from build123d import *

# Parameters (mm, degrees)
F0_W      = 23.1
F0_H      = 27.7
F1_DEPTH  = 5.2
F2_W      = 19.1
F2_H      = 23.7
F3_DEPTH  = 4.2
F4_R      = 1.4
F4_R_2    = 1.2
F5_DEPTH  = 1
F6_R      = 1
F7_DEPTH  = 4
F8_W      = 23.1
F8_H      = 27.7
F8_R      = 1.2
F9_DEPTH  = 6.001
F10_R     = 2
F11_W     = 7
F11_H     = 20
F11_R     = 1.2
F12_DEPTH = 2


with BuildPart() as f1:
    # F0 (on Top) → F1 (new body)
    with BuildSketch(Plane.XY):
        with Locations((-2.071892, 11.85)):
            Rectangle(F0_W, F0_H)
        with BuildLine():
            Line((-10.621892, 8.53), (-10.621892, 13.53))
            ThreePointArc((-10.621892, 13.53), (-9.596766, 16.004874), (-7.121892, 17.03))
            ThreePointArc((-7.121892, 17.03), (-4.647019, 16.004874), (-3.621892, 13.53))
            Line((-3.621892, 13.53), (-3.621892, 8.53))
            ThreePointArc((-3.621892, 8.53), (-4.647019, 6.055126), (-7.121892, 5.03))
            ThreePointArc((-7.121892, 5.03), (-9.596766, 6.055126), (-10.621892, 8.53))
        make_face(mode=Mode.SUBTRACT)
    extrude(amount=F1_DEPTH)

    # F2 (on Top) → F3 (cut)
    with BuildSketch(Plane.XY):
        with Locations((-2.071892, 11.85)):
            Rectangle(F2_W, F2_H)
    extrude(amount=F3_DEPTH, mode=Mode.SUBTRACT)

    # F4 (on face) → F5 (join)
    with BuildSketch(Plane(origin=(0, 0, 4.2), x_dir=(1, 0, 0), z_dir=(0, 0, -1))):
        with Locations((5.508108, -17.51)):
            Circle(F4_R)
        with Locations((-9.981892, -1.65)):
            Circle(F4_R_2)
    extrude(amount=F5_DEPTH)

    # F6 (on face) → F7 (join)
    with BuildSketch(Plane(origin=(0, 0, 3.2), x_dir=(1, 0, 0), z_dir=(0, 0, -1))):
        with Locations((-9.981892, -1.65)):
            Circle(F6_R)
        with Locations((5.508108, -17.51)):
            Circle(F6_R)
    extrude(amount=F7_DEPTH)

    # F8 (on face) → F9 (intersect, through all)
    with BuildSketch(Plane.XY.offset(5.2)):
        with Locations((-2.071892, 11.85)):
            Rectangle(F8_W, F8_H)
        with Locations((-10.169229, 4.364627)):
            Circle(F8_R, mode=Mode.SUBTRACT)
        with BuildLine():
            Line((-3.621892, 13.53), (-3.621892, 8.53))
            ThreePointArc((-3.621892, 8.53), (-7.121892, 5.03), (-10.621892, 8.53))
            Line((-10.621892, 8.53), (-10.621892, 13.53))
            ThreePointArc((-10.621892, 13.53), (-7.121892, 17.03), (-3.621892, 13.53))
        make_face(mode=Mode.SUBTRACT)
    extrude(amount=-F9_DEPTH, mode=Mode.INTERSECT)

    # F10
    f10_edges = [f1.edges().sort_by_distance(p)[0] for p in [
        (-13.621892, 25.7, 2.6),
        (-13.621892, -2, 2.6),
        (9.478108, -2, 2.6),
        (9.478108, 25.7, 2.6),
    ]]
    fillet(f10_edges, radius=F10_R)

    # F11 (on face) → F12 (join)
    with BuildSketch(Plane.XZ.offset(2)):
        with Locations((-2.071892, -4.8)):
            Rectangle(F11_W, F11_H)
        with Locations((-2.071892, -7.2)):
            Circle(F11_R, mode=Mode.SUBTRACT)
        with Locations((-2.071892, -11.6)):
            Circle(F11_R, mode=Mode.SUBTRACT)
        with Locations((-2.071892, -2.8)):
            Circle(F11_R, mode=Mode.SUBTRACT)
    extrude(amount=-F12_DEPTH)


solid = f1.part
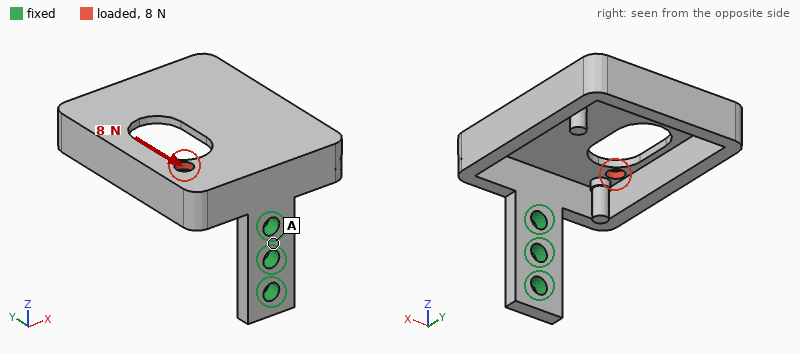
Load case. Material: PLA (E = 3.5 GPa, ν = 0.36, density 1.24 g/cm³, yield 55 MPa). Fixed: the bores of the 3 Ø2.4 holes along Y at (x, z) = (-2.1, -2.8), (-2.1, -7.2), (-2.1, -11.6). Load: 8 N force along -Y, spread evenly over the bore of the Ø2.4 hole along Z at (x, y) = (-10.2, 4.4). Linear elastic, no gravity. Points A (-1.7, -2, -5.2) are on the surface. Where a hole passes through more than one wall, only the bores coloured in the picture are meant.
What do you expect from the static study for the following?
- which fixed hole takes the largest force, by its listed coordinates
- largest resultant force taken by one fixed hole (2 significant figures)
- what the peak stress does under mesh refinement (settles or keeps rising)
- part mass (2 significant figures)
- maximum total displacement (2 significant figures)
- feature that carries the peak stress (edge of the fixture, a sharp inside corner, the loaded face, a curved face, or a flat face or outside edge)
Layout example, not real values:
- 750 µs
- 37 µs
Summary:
- (-2.1, -2.8)
- 10.0 N
- keeps rising
- 1.9 g
- 0.49 mm
- edge of the fixture
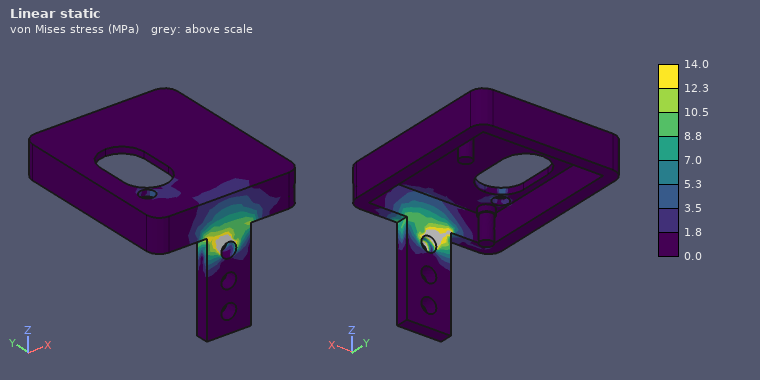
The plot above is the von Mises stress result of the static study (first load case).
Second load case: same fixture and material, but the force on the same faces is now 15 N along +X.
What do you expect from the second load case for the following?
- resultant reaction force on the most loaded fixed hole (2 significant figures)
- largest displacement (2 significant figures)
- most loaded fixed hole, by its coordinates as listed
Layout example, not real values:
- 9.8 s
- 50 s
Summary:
- 23 N
- 0.48 mm
- (-2.1, -2.8)
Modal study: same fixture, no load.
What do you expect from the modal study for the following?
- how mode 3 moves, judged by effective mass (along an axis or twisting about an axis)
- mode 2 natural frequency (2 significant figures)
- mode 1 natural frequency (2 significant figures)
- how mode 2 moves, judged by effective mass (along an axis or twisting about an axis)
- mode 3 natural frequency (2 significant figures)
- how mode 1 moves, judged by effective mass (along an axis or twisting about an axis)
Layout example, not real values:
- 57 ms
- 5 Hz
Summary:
- twisting about Y
- 470 Hz
- 370 Hz
- along X
- 1200 Hz
- along Z
